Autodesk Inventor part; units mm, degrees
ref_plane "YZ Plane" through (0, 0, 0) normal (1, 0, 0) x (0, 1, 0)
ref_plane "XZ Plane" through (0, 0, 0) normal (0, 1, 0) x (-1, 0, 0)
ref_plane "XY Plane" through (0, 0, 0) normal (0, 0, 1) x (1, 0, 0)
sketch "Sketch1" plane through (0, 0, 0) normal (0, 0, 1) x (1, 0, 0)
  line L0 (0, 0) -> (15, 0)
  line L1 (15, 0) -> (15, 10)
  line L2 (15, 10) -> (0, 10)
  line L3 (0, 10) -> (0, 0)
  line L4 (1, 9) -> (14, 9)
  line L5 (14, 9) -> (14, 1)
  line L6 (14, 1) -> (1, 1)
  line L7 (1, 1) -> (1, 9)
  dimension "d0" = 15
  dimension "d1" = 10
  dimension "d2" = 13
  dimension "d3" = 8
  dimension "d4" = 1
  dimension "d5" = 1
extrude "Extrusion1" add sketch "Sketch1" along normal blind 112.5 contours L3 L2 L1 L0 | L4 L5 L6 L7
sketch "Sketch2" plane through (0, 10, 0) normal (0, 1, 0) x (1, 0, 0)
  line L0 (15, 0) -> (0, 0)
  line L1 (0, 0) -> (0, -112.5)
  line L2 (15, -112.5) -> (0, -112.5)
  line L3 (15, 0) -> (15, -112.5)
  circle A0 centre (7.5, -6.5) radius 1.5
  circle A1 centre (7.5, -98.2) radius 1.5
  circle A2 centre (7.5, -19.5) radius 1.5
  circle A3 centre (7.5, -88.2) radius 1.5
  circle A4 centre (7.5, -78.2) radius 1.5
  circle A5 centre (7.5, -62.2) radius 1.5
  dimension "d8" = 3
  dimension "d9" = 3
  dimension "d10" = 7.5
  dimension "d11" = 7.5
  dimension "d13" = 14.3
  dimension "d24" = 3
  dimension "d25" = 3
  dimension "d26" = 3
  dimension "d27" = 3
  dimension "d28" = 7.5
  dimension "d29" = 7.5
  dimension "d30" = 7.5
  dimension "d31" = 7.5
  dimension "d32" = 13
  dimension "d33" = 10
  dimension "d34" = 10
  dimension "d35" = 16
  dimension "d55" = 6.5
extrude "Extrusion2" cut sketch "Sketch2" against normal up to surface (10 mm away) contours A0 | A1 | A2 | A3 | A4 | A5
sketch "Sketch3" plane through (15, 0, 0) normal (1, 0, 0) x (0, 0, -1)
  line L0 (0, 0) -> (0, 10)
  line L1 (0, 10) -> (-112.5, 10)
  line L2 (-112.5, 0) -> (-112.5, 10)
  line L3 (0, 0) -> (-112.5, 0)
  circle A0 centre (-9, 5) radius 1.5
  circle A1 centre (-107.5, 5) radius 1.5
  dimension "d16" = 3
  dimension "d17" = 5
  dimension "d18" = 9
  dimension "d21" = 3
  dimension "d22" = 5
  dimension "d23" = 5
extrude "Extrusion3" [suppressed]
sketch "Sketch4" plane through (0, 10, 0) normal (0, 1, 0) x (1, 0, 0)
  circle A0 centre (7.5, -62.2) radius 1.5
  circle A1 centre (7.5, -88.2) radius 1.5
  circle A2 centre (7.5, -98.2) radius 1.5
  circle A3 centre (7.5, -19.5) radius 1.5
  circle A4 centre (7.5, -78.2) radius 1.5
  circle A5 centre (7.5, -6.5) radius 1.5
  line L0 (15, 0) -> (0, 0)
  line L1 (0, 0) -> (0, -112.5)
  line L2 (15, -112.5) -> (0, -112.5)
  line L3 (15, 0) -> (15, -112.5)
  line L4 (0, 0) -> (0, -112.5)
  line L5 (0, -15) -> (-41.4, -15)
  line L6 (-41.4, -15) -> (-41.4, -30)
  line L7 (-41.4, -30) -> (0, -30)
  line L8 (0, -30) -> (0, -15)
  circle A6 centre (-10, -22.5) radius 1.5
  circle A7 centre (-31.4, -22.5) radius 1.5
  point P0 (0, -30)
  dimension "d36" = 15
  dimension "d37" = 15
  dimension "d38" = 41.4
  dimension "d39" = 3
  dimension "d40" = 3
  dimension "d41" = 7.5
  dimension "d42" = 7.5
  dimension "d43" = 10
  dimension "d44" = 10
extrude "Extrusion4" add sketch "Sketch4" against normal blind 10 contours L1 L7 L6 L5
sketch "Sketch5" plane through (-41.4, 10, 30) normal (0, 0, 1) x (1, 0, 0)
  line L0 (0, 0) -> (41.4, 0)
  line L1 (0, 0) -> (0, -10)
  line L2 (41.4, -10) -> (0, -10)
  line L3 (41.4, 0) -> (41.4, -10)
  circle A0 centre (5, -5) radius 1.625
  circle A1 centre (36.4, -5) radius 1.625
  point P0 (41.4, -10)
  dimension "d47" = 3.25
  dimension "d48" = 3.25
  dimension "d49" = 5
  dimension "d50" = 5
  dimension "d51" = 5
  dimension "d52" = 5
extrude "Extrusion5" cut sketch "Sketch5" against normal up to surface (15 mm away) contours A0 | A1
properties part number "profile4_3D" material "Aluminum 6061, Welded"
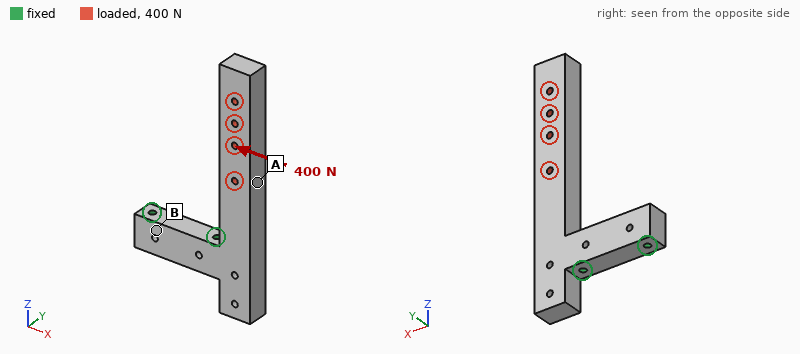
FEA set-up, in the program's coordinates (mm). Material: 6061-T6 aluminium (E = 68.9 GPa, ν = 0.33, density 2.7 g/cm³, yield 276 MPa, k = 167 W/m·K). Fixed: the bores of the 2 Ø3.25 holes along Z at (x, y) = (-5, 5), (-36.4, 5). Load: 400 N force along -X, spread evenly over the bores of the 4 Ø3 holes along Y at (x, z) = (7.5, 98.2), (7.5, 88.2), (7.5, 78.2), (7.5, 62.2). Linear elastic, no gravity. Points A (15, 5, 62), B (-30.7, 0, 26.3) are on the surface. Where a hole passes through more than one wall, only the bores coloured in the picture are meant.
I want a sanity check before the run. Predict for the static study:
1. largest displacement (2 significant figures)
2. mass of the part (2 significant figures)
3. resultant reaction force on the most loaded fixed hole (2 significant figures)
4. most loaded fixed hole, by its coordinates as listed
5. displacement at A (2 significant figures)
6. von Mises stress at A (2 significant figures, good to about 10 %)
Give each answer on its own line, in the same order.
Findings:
0.36 mm
60 g
390 N
(-5, 5)
0.12 mm
21 MPa
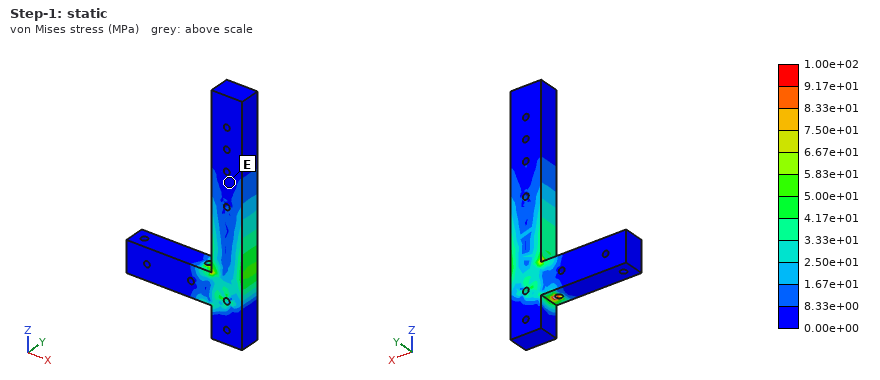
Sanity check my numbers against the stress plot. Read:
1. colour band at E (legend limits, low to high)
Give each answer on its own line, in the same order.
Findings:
0.00e+00 to 8.33e+00 MPa
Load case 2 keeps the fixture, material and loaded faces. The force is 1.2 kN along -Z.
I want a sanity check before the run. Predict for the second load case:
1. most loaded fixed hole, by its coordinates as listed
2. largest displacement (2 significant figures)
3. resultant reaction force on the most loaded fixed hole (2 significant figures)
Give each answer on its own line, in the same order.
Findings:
(-5, 5)
62 µm
1.2 kN
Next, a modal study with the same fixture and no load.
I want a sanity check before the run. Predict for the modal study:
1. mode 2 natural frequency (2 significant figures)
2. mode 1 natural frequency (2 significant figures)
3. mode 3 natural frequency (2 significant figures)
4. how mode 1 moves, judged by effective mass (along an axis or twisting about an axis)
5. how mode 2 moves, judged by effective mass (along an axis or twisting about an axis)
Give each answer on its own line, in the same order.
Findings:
1300 Hz
890 Hz
4900 Hz
along Y
along X
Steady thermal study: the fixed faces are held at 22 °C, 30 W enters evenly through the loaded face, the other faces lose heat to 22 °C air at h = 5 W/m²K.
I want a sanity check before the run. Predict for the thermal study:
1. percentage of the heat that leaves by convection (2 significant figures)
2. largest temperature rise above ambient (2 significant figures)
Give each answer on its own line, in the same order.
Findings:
4.2 %
77 K
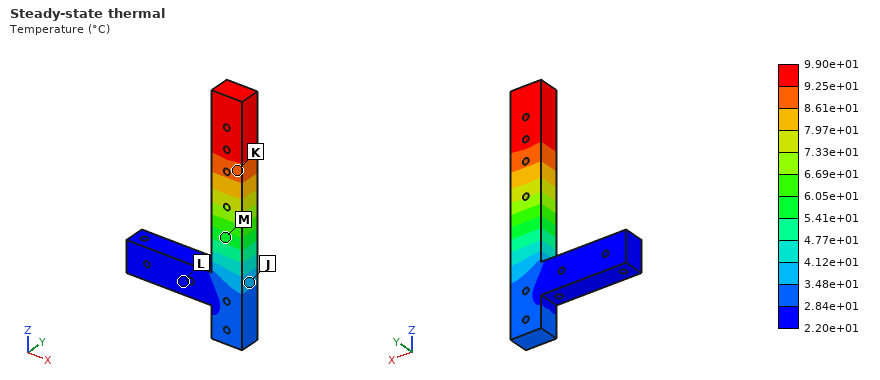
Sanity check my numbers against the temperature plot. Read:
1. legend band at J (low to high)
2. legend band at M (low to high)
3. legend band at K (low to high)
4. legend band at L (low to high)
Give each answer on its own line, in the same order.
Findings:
3.48e+01 to 4.12e+01 °C
5.41e+01 to 6.05e+01 °C
8.61e+01 to 9.25e+01 °C
2.20e+01 to 2.84e+01 °C
